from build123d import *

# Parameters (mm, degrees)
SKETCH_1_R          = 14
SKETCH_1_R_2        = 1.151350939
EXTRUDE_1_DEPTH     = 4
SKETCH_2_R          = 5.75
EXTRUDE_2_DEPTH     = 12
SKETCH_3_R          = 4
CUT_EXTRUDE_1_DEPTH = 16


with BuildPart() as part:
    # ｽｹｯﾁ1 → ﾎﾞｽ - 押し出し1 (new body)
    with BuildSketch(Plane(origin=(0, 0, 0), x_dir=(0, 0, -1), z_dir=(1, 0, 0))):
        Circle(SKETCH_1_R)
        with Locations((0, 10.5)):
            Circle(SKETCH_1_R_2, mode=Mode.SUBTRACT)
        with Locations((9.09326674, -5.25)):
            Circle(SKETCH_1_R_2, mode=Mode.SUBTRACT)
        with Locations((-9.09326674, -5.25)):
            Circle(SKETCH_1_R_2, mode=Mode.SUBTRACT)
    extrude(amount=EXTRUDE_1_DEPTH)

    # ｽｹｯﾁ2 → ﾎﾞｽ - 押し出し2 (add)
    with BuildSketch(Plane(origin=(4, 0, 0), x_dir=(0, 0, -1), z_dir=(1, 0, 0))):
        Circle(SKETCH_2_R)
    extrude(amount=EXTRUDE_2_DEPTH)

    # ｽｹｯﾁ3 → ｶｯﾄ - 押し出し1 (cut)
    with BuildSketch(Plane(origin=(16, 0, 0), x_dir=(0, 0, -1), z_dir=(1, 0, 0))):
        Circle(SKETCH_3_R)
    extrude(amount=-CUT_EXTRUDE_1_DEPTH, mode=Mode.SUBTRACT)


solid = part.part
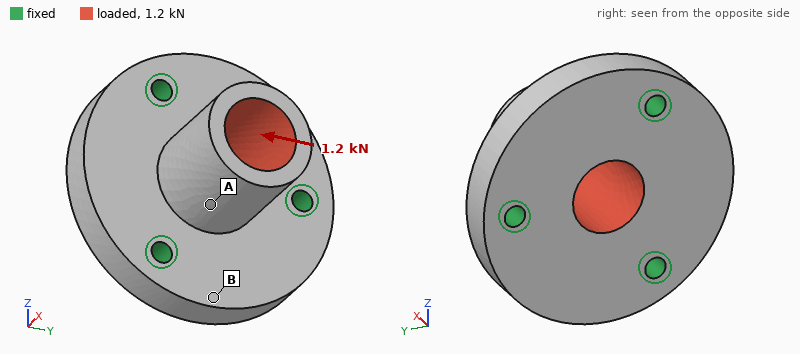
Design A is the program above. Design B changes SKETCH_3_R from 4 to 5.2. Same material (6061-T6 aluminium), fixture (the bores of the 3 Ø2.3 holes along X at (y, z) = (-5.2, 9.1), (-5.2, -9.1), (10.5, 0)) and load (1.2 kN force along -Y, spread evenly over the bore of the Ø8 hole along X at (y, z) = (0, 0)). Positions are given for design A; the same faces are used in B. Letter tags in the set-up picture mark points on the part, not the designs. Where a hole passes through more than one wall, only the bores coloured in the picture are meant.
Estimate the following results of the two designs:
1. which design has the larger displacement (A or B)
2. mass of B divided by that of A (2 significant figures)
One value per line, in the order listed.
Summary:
B
0.81
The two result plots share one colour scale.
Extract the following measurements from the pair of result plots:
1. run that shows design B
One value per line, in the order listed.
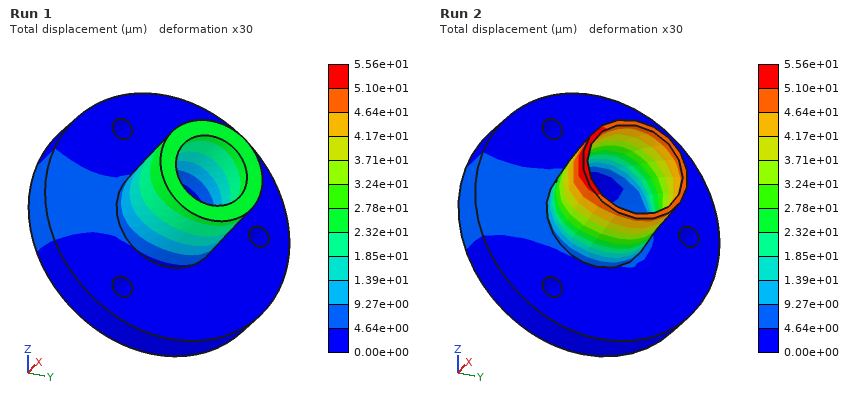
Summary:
Run 2
